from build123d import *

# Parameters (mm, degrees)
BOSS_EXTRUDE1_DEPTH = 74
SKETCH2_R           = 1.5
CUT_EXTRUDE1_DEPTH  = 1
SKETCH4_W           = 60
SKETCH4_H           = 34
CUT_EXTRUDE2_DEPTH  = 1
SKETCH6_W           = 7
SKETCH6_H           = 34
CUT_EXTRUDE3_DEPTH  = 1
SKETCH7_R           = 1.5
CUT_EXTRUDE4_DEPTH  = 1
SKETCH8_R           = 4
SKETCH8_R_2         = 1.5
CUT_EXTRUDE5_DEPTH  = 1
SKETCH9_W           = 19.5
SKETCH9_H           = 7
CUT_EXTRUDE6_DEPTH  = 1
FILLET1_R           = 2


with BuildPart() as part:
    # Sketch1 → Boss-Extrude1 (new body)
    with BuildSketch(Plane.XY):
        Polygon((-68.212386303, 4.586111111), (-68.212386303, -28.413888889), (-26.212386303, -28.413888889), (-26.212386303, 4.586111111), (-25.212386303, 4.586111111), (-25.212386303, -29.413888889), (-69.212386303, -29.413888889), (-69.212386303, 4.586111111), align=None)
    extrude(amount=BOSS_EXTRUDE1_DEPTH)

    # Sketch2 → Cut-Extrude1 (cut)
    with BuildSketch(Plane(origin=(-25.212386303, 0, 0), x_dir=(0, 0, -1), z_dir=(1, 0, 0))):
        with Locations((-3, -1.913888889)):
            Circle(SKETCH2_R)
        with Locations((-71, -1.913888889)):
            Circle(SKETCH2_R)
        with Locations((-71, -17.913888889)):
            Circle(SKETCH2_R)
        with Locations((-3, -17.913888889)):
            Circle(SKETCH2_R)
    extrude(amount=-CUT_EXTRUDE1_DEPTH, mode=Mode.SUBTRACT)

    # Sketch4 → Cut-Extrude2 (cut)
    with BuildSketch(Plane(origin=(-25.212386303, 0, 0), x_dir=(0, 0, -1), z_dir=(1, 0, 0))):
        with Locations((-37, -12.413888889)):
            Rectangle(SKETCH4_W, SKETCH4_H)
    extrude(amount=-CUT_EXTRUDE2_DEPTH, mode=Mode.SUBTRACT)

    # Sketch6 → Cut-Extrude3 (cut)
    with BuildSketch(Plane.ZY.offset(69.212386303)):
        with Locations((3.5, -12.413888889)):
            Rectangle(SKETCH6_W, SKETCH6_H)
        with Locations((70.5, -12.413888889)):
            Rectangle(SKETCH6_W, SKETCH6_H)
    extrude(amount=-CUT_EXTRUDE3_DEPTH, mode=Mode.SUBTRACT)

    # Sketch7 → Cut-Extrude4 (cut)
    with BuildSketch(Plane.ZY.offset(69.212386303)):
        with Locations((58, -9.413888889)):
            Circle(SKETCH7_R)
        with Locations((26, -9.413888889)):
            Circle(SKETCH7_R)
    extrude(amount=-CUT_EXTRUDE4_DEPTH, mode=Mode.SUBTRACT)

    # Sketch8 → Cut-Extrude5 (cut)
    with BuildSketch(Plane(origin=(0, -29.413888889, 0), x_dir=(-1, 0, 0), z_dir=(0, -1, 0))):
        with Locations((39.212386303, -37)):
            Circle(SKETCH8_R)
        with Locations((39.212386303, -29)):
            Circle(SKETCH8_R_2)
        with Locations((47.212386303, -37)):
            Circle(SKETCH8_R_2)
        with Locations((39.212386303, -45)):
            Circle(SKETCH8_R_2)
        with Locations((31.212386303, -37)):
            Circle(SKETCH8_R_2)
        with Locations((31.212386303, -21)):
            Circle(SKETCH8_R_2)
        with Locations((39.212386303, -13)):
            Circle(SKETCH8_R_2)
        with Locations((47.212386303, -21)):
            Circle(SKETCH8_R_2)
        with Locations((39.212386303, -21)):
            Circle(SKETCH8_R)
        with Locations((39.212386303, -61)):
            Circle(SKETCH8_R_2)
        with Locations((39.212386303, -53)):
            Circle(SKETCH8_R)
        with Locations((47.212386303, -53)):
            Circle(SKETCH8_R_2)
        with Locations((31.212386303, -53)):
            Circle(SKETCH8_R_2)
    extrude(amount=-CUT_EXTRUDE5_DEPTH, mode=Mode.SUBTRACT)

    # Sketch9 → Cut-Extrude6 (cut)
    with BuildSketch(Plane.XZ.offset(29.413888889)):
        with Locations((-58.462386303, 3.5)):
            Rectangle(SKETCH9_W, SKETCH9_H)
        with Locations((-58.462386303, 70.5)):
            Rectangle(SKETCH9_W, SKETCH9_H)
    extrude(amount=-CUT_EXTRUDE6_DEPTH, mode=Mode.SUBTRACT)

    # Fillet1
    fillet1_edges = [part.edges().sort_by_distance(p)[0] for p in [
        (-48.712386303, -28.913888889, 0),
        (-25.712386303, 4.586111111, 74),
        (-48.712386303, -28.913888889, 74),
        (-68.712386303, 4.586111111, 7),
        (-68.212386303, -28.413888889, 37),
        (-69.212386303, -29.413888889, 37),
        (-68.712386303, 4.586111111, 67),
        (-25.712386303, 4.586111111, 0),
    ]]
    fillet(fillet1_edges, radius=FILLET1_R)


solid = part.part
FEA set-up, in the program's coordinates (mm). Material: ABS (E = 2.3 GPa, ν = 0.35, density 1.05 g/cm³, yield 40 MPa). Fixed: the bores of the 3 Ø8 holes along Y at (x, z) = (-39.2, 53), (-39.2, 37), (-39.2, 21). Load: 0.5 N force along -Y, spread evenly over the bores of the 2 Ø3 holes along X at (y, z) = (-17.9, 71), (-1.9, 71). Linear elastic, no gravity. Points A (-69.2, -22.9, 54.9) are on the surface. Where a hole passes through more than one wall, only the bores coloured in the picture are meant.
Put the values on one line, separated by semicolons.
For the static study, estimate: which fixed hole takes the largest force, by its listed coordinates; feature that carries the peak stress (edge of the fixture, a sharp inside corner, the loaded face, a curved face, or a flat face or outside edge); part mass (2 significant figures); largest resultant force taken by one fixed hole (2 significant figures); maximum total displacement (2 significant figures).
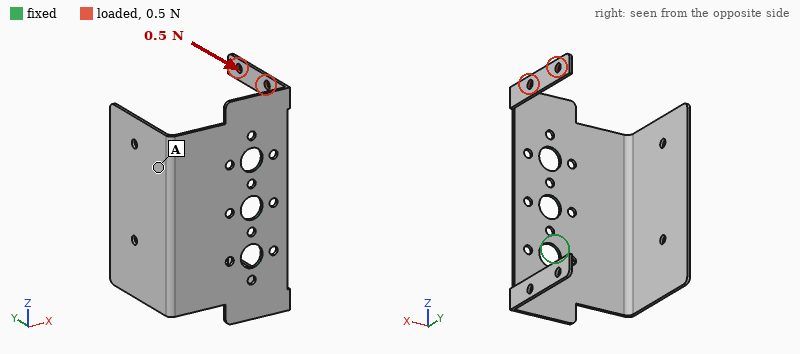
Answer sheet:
(-39.2, 53); a curved face; 5.3 g; 0.57 N; 0.96 mm
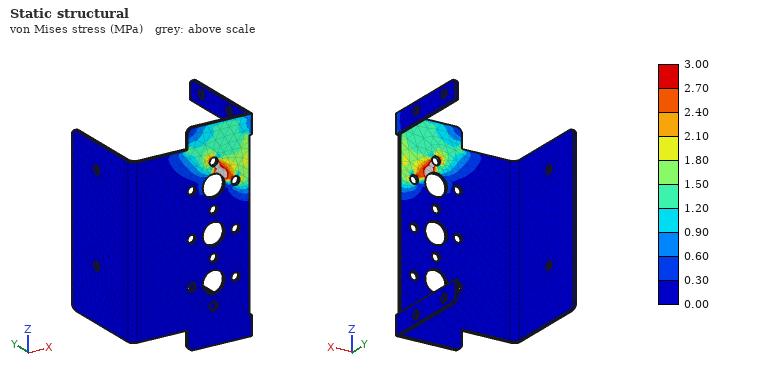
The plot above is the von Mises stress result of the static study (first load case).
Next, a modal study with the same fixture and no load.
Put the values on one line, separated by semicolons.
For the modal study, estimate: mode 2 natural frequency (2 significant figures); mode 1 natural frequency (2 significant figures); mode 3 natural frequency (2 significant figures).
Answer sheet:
150 Hz; 92 Hz; 160 Hz
